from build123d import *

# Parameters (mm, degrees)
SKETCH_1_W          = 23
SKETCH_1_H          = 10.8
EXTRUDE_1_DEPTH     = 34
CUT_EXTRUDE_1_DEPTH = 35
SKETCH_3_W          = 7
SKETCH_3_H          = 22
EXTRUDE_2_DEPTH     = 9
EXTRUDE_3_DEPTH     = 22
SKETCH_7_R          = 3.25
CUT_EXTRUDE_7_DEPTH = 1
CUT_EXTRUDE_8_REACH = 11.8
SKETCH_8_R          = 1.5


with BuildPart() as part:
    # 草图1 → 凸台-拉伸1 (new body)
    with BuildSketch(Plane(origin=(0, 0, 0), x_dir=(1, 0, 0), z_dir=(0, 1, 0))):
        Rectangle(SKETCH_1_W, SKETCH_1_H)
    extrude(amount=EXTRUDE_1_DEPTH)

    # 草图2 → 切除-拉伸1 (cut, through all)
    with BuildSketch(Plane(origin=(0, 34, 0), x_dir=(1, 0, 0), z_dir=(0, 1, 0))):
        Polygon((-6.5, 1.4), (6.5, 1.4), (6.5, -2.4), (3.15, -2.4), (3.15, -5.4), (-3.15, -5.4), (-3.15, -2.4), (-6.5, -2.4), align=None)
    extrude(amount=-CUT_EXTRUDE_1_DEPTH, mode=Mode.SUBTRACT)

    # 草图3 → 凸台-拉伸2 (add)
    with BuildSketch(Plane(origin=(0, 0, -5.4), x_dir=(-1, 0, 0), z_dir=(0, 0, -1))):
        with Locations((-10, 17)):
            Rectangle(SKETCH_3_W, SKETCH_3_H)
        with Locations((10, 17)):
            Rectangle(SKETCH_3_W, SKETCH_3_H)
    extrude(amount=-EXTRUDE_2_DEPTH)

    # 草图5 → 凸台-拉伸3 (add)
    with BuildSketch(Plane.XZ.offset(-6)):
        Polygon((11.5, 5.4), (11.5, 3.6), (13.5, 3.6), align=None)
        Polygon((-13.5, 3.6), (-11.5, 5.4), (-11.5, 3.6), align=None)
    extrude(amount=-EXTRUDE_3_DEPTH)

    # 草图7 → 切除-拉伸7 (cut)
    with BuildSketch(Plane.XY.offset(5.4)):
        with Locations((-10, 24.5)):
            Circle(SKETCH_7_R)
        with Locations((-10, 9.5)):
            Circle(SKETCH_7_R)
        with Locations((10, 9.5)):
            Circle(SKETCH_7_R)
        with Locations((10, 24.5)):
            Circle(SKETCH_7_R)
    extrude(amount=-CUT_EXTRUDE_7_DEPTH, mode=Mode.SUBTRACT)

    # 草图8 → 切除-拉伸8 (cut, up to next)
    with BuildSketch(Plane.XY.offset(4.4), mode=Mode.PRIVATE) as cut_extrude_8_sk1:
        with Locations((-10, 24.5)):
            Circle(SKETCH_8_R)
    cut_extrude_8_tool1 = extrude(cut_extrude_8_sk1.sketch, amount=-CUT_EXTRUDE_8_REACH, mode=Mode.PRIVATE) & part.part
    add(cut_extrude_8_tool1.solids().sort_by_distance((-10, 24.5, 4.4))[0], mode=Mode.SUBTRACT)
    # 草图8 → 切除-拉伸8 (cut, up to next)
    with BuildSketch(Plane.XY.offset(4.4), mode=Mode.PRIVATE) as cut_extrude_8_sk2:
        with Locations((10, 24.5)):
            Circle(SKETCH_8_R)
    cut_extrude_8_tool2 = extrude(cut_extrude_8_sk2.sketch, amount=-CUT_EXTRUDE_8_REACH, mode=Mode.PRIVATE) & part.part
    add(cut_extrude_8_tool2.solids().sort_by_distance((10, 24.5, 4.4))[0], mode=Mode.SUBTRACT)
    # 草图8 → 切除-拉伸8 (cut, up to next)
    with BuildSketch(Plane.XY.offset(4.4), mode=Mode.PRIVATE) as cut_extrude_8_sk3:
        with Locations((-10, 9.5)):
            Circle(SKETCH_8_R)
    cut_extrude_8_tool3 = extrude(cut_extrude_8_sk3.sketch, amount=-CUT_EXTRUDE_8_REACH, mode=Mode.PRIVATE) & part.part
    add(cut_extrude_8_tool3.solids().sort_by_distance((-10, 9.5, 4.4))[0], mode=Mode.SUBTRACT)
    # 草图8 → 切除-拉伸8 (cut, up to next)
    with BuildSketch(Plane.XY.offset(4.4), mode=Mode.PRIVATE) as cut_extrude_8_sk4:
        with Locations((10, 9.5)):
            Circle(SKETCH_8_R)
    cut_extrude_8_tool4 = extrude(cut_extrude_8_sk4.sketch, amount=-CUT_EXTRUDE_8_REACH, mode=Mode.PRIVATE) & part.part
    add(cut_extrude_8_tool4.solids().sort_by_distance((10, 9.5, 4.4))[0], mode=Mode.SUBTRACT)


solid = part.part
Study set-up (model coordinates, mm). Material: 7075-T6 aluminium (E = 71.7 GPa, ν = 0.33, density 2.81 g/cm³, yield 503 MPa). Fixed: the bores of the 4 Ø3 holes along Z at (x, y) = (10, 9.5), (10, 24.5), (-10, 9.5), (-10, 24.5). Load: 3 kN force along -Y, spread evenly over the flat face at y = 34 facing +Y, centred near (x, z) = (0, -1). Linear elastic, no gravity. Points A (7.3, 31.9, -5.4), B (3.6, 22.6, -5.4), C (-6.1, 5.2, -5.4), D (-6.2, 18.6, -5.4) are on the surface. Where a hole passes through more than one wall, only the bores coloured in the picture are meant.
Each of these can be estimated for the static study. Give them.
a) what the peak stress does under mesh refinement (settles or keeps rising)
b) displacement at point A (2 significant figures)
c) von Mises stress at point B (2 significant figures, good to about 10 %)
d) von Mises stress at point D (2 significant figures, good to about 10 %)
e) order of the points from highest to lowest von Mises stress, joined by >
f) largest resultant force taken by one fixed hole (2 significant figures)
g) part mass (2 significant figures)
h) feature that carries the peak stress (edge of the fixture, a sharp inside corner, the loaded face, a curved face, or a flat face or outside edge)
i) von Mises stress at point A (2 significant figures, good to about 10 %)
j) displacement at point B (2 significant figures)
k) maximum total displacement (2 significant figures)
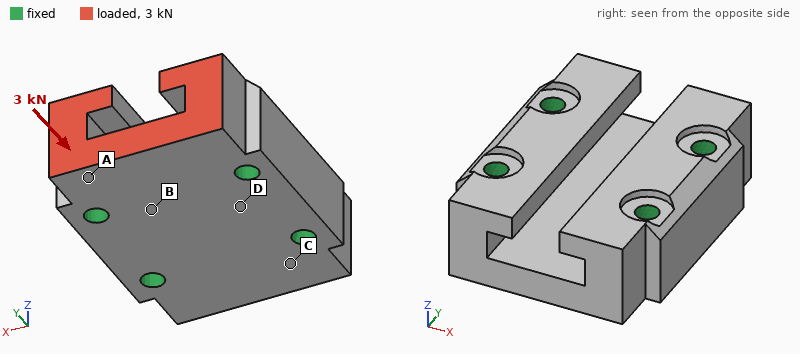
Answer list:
keeps rising
2.1 µm
10 MPa
7.6 MPa
A > B > D > C
1.3 kN
19 g
edge of the fixture
17 MPa
1.3 µm
4.4 µm
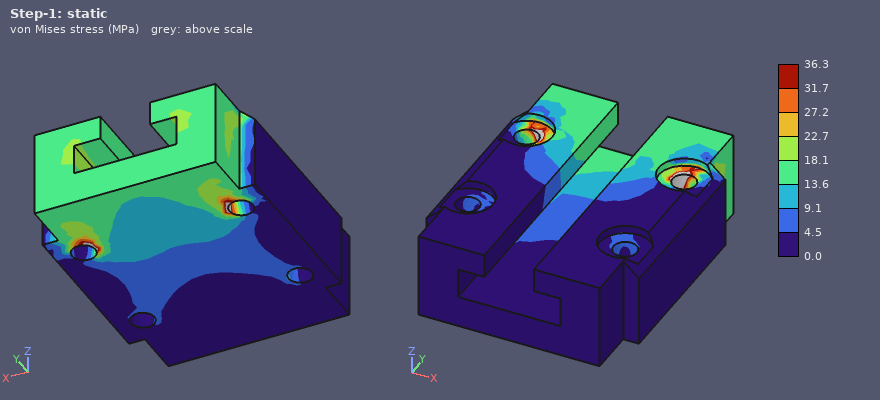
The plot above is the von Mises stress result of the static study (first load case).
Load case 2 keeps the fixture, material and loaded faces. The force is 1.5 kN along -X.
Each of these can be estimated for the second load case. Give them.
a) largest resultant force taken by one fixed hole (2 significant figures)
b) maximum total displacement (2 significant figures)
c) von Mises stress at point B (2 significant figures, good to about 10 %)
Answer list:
960 N
11 µm
6.3 MPa
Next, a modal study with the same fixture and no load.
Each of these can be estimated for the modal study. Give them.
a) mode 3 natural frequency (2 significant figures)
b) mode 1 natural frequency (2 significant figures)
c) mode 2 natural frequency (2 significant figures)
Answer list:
53 kHz
42 kHz
42 kHz
